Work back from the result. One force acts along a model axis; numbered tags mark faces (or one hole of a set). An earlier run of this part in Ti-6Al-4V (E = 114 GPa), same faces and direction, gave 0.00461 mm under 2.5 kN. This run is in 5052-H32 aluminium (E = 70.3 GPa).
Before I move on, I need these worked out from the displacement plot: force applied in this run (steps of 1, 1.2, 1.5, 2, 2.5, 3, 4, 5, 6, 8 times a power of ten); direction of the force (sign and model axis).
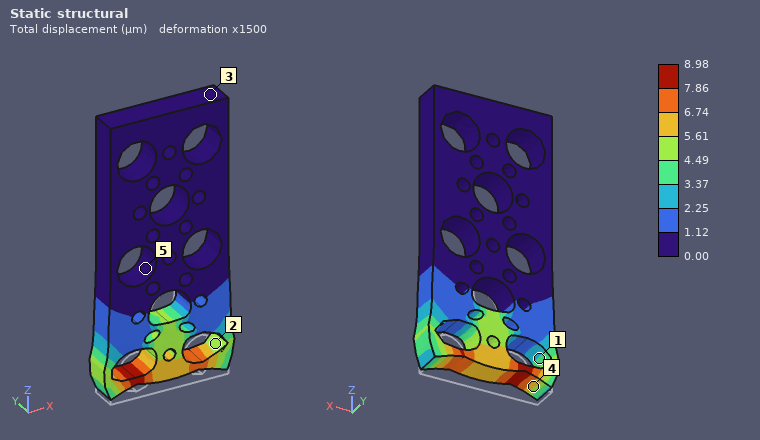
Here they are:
3 kN
+Z
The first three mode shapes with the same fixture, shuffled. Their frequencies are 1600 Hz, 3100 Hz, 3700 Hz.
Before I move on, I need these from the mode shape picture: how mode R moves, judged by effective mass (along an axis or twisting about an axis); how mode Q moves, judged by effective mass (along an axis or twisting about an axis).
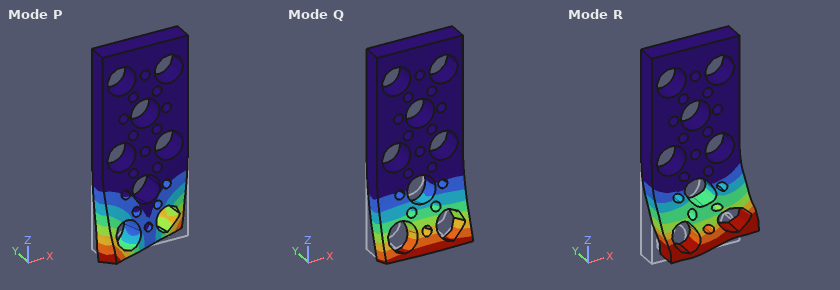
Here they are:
along X
along Y
